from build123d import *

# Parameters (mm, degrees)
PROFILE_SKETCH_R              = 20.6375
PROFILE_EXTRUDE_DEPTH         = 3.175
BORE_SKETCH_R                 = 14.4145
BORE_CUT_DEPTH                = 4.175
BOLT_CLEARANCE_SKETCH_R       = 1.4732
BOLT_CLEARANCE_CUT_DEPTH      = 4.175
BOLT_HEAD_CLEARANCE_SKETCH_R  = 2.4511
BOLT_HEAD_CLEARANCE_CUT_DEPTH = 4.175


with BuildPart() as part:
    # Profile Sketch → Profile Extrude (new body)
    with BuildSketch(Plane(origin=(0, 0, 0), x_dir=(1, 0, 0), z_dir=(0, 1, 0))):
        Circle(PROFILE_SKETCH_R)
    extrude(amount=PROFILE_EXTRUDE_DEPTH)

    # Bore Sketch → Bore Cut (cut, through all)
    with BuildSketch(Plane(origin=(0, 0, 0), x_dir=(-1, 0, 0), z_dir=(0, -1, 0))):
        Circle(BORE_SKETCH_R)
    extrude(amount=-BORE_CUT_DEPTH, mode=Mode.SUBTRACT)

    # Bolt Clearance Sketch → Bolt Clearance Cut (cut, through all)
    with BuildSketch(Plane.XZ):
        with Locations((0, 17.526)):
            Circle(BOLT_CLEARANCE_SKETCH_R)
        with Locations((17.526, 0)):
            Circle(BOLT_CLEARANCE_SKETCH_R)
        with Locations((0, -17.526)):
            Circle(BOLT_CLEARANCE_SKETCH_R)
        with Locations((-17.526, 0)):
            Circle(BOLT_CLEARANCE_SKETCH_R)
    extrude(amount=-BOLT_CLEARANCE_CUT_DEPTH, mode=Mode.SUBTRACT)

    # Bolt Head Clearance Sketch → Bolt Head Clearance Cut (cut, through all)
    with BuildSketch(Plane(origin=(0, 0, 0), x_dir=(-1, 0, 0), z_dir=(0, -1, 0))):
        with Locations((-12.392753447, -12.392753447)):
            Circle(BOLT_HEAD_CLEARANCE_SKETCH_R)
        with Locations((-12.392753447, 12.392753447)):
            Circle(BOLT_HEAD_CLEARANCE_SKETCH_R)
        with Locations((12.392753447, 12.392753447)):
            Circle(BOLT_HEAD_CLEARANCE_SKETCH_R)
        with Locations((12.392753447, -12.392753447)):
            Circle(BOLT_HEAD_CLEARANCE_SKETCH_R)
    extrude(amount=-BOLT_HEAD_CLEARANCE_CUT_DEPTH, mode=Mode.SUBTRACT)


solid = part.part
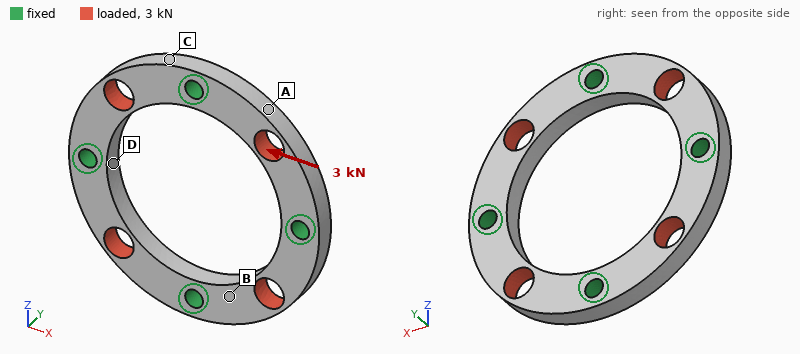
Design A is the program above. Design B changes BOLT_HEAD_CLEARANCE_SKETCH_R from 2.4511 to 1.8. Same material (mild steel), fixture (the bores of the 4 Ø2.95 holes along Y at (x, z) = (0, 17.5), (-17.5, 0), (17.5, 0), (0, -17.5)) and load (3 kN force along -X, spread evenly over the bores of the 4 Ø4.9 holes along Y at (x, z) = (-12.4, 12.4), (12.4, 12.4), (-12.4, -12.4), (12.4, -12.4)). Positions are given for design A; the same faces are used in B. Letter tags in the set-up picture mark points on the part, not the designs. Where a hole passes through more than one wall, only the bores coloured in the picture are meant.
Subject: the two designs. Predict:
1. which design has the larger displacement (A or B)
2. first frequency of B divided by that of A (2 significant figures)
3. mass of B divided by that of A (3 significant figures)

A
0.97
1.06
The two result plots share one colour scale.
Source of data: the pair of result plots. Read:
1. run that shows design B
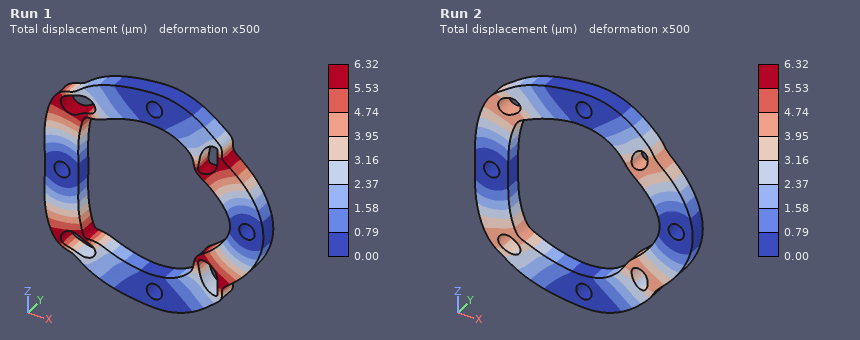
Run 2
